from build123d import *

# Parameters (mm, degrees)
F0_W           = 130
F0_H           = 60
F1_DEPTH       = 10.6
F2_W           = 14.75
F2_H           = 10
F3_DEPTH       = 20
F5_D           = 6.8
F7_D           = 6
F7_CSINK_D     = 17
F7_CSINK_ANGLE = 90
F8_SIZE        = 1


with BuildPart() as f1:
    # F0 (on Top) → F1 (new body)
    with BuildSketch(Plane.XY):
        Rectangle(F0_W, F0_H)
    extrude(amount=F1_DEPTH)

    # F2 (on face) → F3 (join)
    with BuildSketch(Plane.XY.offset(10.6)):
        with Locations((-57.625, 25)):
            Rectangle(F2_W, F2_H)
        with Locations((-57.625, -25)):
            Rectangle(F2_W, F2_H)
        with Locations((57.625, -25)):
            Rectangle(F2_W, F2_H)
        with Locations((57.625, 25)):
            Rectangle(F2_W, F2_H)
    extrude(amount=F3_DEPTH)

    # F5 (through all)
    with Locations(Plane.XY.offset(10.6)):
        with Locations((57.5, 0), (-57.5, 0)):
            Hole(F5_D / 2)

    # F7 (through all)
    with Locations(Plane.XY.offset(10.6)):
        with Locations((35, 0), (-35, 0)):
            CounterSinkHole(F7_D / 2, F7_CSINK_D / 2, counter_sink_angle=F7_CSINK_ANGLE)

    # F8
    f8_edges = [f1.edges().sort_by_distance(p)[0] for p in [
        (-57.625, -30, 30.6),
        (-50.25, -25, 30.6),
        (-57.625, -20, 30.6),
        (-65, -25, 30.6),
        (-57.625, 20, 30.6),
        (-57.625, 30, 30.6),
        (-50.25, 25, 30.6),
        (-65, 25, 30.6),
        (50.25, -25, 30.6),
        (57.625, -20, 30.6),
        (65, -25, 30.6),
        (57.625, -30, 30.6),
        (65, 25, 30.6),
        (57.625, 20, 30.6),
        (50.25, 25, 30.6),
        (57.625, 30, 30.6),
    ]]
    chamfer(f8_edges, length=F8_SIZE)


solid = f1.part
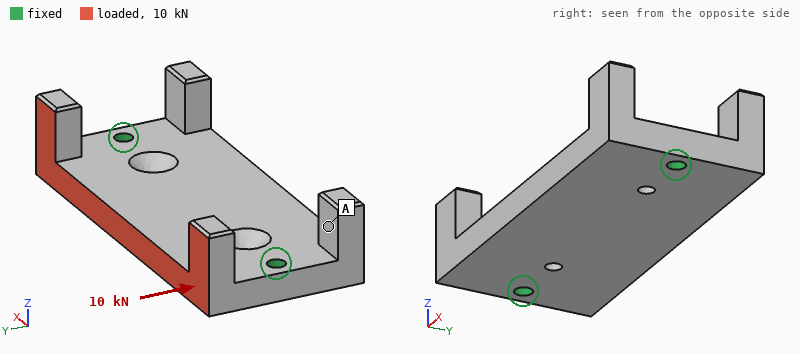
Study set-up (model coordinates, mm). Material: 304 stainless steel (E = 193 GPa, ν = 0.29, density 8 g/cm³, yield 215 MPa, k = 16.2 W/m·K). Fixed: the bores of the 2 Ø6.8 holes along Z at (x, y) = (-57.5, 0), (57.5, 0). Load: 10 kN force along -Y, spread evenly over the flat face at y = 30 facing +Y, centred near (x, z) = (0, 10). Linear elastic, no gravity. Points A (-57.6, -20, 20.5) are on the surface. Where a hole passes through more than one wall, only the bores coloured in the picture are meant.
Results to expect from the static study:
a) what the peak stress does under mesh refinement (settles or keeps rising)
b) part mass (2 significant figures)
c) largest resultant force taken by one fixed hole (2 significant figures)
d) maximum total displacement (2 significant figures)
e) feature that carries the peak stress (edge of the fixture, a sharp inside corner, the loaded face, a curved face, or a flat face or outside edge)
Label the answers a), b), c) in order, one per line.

a) keeps rising
b) 740 g
c) 5.0 kN
d) 42 µm
e) edge of the fixture
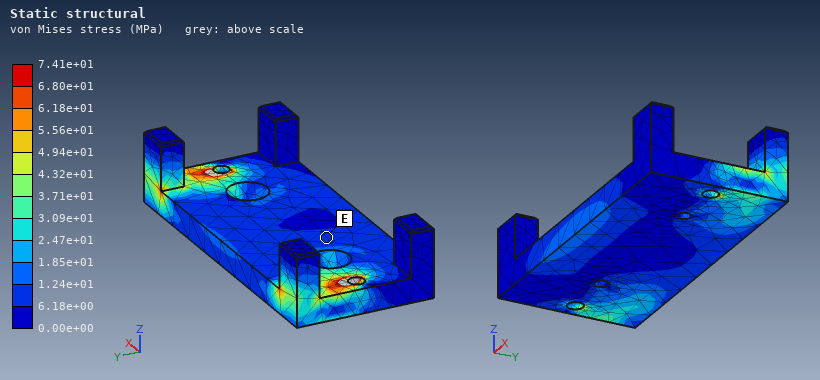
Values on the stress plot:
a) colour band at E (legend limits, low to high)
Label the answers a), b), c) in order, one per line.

a) 6.18e+00 to 1.24e+01 MPa
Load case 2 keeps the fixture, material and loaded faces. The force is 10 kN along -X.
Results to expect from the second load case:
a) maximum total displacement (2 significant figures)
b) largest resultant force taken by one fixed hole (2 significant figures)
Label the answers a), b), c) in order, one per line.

a) 29 µm
b) 5.6 kN
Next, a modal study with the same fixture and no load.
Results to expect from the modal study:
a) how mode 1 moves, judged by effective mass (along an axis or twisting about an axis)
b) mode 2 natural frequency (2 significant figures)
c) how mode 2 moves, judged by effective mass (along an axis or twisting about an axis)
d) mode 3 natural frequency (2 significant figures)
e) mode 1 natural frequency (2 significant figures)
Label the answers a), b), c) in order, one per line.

a) along Z
b) 3300 Hz
c) twisting about X
d) 5300 Hz
e) 3100 Hz
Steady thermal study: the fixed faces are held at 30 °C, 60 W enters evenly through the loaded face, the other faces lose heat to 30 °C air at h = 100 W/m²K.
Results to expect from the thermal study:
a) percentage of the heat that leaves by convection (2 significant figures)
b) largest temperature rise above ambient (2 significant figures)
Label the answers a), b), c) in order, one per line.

a) 73 %
b) 73 K
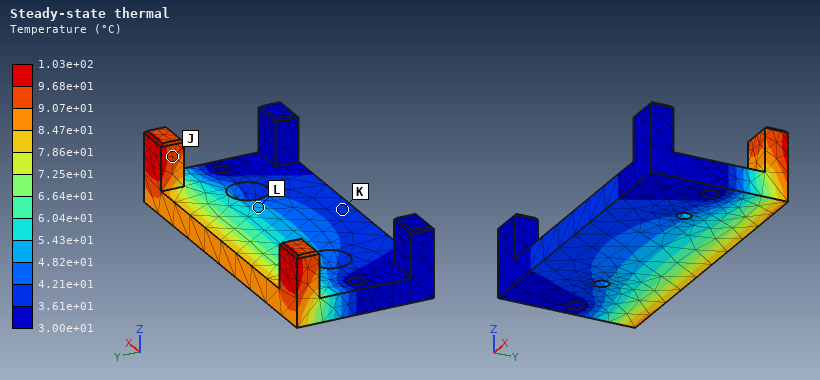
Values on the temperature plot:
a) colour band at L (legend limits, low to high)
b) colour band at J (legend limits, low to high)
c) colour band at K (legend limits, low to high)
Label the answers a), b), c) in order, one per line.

a) 4.82e+01 to 5.43e+01 °C
b) 9.07e+01 to 9.68e+01 °C
c) 3.61e+01 to 4.21e+01 °C
